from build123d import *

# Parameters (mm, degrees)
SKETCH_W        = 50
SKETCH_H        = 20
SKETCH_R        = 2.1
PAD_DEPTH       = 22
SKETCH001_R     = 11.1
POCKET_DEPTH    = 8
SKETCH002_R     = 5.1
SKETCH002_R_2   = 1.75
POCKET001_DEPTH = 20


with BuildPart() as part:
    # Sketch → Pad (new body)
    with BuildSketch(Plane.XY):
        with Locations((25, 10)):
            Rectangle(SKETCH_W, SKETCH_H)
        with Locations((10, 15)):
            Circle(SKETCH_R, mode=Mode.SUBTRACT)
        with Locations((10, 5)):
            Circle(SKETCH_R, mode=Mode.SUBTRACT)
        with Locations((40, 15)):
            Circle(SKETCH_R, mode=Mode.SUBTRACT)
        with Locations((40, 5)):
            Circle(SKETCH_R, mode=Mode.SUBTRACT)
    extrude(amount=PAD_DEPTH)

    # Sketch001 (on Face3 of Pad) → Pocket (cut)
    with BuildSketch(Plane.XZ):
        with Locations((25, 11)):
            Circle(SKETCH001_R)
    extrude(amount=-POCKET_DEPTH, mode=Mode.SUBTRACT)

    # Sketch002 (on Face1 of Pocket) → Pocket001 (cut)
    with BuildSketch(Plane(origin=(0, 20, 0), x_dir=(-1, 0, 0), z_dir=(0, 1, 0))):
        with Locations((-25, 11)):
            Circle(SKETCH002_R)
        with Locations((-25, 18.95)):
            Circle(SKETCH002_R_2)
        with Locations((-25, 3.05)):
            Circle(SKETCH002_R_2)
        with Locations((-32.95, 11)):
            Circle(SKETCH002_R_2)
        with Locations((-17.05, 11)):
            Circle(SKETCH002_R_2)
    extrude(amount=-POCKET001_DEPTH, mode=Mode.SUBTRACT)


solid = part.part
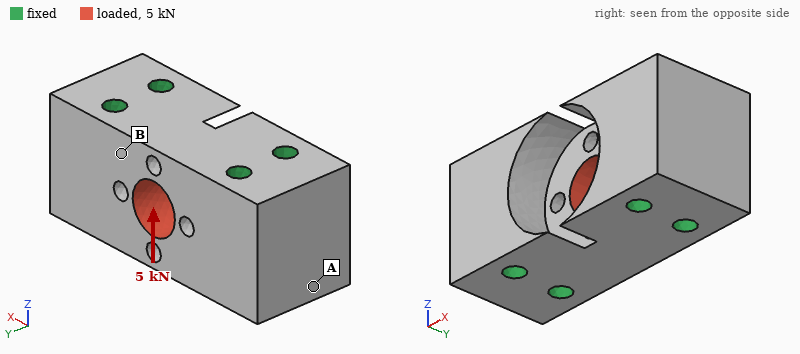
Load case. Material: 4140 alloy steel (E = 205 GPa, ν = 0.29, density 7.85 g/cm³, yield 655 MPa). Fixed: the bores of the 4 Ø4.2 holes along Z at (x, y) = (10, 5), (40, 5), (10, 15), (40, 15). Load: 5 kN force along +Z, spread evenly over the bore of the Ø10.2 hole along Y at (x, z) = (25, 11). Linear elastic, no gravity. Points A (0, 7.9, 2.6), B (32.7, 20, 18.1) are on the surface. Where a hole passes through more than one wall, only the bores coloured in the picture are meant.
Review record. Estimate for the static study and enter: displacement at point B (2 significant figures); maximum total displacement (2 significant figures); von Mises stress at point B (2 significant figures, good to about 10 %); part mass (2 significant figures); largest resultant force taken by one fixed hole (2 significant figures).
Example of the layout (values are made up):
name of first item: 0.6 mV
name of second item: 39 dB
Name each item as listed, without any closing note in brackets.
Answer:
displacement at point B: 1.1 µm
maximum total displacement: 3.0 µm
von Mises stress at point B: 21 MPa
part mass: 130 g
largest resultant force taken by one fixed hole: 1.9 kN
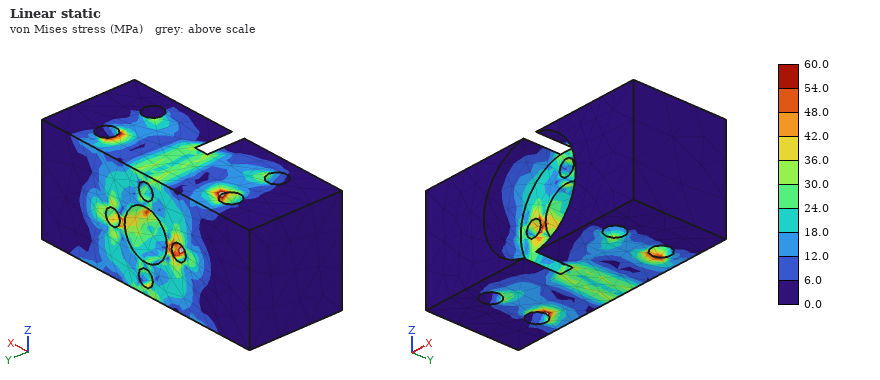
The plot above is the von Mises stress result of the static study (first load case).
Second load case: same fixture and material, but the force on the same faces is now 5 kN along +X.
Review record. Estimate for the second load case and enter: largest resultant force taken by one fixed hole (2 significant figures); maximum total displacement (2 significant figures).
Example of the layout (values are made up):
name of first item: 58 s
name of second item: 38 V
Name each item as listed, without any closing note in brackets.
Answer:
largest resultant force taken by one fixed hole: 2.0 kN
maximum total displacement: 1.1 µm
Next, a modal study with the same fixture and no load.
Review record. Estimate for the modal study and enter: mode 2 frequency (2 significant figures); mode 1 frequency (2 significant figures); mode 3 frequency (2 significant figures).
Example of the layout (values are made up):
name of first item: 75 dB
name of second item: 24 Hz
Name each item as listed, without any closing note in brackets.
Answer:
mode 2 frequency: 55 kHz
mode 1 frequency: 55 kHz
mode 3 frequency: 60 kHz
